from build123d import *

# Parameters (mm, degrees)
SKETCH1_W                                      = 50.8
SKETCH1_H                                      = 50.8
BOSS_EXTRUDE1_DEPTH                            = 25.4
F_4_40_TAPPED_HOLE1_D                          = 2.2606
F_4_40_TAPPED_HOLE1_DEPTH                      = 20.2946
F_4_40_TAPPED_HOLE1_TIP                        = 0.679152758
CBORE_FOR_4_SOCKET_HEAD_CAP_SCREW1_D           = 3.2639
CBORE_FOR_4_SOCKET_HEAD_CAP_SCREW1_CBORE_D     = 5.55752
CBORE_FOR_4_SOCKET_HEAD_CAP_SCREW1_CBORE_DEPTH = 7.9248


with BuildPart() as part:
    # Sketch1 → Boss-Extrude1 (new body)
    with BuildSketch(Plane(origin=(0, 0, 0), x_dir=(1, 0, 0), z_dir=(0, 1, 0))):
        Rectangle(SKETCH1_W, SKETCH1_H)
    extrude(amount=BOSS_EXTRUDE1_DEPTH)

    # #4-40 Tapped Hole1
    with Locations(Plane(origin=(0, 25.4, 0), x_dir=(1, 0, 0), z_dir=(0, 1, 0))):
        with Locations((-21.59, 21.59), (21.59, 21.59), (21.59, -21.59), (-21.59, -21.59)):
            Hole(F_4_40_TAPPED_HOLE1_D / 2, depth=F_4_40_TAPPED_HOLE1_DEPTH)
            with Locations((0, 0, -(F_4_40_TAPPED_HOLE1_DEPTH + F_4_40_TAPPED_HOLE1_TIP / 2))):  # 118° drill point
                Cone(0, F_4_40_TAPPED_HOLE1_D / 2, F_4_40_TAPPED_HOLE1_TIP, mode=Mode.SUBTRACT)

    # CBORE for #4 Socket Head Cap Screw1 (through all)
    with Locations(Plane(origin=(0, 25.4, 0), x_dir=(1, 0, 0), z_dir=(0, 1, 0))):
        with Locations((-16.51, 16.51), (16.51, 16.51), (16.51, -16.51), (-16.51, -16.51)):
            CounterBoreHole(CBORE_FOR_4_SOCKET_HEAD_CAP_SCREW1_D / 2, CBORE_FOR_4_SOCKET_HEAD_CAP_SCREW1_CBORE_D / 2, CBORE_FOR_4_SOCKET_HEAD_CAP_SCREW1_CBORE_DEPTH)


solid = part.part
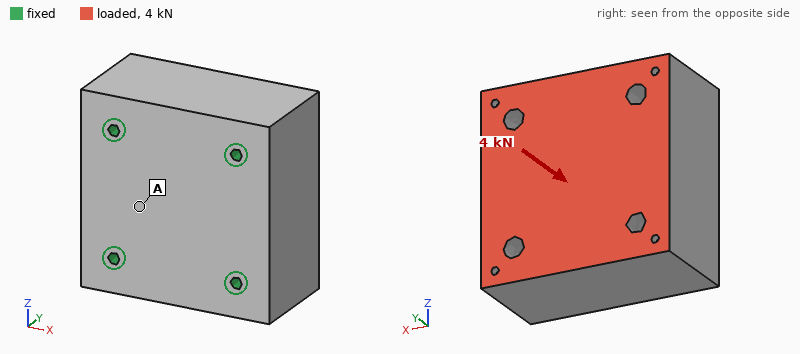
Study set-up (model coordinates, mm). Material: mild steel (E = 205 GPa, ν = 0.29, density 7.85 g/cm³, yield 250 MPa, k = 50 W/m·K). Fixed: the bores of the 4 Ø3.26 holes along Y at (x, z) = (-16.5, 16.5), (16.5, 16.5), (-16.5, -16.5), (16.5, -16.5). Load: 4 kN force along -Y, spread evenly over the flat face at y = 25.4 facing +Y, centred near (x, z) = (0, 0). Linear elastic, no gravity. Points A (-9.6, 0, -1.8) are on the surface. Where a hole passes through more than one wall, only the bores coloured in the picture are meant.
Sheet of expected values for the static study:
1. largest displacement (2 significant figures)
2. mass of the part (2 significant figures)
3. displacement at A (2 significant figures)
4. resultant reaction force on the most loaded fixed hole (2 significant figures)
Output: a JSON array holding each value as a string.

["0.40 µm", "500 g", "0.29 µm", "1.0 kN"]
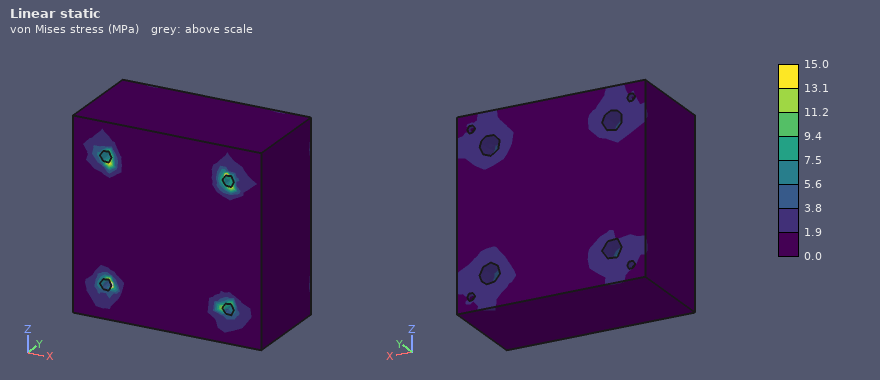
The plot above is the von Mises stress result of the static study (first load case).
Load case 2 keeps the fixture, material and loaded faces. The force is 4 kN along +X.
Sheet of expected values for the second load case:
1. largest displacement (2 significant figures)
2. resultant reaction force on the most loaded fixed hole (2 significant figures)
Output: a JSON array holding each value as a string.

["0.99 µm", "1.2 kN"]
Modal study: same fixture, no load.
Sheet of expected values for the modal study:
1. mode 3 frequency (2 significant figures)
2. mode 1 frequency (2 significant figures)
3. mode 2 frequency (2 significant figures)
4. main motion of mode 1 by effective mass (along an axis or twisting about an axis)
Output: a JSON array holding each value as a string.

["30 kHz", "28 kHz", "30 kHz", "along Y"]
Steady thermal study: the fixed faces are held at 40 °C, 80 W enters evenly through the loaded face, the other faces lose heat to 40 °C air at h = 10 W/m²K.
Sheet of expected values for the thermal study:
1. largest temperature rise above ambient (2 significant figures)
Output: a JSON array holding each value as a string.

["16 K"]
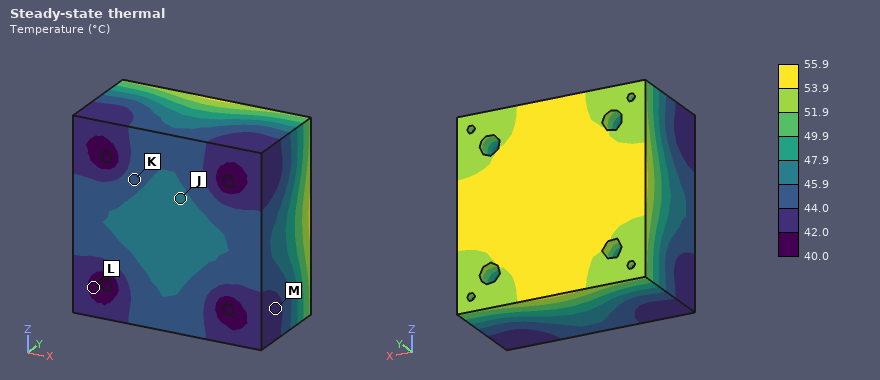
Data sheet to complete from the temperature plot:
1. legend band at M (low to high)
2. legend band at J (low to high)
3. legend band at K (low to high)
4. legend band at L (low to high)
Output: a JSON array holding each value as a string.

["42.0 to 44.0 °C", "45.9 to 47.9 °C", "44.0 to 45.9 °C", "40.0 to 42.0 °C"]
